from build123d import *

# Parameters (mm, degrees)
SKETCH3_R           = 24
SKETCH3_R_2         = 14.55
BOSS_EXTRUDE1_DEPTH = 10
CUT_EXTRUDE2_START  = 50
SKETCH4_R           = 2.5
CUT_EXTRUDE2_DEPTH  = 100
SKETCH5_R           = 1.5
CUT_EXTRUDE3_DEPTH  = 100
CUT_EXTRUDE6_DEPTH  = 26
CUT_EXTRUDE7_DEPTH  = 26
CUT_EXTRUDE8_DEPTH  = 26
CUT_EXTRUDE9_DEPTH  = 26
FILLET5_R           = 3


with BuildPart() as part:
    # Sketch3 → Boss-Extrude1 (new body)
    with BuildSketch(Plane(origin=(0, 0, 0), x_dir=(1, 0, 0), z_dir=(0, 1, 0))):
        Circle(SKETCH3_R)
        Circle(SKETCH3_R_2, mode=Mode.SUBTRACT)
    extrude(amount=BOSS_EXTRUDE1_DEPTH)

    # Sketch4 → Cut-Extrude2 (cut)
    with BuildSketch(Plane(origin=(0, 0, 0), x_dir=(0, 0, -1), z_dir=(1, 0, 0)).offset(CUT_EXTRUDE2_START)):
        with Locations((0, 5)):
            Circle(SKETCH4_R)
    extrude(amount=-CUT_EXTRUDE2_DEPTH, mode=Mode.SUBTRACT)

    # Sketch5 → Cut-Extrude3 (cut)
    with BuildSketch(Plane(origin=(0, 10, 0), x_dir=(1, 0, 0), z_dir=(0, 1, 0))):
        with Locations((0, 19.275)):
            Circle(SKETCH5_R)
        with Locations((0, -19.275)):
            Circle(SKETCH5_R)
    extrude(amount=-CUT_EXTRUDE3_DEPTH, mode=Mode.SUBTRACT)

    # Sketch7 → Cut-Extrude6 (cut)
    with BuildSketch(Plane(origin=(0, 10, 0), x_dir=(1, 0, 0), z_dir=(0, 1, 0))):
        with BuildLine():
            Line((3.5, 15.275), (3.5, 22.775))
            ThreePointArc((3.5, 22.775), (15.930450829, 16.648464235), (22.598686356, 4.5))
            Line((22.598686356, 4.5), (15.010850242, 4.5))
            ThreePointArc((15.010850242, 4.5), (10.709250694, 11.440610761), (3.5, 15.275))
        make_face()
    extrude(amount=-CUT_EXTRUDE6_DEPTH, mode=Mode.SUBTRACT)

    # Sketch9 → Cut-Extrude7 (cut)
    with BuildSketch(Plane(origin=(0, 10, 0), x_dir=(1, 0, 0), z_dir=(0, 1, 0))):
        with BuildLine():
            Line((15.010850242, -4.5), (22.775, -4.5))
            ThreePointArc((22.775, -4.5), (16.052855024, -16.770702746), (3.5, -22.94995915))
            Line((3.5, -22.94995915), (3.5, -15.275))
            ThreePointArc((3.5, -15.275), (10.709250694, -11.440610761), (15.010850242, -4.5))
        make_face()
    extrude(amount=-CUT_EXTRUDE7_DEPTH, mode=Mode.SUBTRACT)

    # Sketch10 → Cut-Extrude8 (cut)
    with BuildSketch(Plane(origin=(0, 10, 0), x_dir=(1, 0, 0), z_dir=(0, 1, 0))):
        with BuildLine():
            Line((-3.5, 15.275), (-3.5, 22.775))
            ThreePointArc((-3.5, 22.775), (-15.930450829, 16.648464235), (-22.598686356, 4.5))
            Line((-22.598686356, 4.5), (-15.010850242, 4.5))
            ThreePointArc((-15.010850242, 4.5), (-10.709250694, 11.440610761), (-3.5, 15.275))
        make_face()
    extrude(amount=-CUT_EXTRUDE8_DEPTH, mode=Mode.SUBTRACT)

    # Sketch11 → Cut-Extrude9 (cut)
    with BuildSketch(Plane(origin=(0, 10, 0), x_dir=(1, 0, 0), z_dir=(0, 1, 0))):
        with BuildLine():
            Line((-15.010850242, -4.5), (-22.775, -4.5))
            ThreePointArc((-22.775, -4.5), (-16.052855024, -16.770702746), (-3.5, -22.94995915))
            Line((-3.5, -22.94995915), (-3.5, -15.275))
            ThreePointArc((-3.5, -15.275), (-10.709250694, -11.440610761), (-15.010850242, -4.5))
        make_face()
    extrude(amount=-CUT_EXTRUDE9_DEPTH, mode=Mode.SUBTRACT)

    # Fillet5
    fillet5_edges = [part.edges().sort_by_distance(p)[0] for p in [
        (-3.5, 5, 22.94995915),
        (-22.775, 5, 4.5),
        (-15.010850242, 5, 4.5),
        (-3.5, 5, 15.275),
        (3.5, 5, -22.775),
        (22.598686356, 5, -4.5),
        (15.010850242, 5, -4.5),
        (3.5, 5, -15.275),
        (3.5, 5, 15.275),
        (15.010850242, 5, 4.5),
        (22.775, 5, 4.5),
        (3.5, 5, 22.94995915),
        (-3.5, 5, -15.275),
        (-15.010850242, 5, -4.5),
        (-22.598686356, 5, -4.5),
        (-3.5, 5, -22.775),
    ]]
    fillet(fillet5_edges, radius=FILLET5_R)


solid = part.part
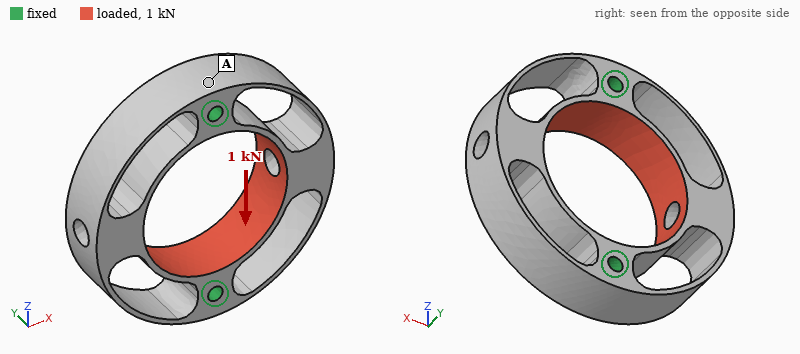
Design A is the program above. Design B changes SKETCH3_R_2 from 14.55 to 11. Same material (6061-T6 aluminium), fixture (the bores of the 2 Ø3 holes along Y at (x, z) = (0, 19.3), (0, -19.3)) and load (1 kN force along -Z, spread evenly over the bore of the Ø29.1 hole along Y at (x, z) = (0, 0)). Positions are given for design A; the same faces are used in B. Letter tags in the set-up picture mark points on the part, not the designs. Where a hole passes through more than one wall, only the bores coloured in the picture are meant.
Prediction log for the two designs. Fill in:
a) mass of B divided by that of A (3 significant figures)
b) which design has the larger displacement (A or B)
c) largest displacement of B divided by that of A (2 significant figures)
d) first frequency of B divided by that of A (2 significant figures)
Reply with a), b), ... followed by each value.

a) 1.59
b) A
c) 0.035
d) 1.5
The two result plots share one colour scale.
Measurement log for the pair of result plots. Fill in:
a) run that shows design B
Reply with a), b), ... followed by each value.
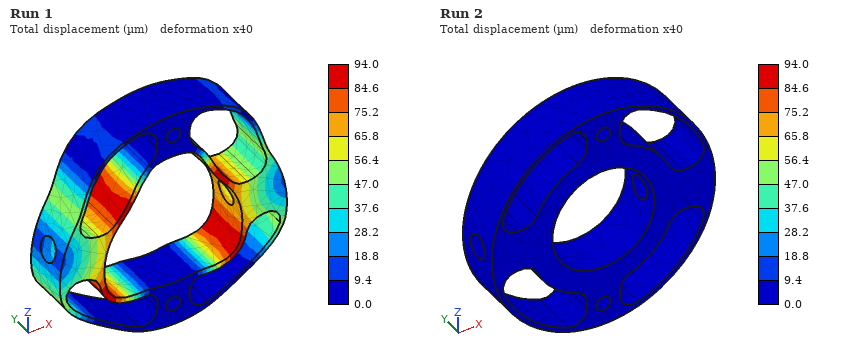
a) Run 2
